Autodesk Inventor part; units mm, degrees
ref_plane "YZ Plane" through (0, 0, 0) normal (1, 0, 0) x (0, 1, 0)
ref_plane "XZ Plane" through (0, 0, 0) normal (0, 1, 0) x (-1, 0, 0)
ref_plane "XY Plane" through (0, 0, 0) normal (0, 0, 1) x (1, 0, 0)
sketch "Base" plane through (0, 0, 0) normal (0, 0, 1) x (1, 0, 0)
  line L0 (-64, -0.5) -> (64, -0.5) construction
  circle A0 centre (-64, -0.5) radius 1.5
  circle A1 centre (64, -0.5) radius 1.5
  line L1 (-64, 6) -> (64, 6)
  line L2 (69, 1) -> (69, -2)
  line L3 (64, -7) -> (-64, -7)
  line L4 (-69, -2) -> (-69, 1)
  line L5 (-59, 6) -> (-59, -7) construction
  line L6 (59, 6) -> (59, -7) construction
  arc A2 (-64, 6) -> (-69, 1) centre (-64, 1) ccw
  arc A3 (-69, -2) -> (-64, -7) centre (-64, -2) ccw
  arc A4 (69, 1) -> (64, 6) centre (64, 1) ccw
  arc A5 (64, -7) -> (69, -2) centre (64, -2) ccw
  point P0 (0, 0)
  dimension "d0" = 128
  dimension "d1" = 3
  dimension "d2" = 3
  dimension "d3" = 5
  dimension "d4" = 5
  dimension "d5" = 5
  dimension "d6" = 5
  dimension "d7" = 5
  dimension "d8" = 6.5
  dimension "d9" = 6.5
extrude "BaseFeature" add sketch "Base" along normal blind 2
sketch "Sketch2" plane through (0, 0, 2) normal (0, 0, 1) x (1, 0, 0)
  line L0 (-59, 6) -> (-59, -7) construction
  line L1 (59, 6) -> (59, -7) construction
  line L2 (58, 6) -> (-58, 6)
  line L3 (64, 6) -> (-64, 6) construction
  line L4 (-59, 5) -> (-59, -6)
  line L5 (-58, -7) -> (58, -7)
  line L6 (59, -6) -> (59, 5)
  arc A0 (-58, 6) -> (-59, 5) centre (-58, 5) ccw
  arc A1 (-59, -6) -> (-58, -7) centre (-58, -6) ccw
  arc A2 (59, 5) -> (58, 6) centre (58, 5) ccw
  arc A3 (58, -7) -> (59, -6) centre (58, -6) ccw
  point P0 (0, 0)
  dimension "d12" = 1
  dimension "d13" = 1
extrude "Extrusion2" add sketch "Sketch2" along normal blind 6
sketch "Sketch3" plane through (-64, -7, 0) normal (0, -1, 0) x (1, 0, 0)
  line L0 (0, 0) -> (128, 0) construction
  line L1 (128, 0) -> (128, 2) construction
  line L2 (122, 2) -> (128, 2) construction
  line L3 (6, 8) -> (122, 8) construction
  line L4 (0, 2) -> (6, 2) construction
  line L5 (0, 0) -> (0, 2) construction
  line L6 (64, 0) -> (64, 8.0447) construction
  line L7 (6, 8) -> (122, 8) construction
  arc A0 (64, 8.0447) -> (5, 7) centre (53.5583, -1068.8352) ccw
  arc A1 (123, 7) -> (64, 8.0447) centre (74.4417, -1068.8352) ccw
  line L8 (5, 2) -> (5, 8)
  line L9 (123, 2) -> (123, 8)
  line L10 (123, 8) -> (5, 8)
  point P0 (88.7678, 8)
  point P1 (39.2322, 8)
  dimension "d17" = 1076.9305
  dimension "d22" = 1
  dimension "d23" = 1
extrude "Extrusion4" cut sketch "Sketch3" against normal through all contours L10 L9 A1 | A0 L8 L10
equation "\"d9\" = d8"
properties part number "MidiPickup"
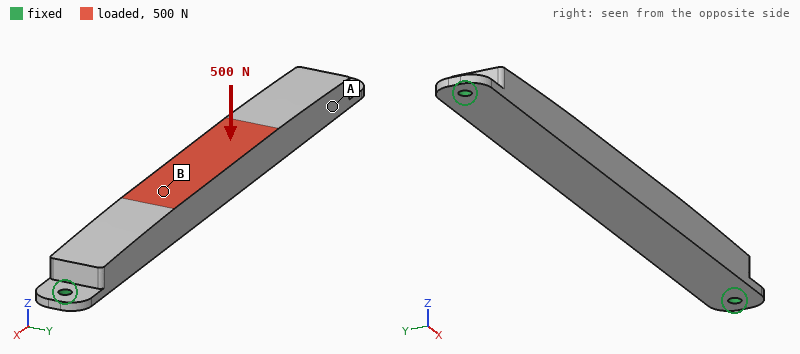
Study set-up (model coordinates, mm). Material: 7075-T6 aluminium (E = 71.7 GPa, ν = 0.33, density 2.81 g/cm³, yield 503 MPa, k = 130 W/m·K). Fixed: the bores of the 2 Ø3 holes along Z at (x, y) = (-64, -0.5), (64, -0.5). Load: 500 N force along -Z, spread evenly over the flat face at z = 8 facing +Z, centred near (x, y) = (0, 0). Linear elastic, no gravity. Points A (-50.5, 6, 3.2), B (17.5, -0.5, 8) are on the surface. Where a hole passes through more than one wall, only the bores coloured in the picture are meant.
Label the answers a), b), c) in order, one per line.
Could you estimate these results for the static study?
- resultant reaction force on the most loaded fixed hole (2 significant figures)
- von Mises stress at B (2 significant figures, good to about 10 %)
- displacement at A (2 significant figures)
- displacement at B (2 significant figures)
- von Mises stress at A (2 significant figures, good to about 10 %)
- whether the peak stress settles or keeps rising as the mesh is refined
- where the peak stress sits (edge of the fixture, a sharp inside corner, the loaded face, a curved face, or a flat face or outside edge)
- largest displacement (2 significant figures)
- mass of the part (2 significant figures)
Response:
a) 1.2 kN
b) 58 MPa
c) 0.062 mm
d) 0.23 mm
e) 17 MPa
f) keeps rising
g) edge of the fixture
h) 0.26 mm
i) 35 g
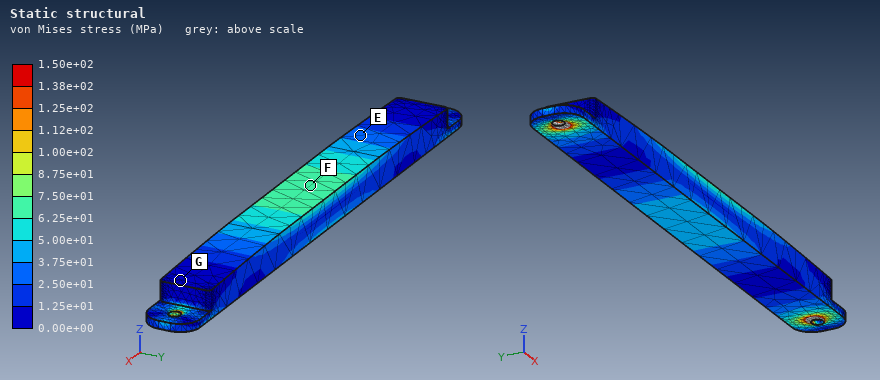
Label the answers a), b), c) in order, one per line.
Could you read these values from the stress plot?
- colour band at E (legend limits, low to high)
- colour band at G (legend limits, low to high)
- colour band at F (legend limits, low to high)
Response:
a) 2.50e+01 to 3.75e+01 MPa
b) 0.00e+00 to 1.25e+01 MPa
c) 6.25e+01 to 7.50e+01 MPa
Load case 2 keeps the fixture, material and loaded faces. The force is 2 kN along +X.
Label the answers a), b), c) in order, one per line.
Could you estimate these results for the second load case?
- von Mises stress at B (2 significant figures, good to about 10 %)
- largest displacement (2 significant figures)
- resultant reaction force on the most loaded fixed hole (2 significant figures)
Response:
a) 14 MPa
b) 14 µm
c) 1.0 kN
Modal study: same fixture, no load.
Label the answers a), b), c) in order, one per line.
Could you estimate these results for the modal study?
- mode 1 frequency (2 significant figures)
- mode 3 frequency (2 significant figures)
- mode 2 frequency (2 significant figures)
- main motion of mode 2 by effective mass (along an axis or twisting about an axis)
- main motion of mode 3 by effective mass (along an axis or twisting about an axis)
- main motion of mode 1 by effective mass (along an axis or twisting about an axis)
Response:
a) 1600 Hz
b) 4300 Hz
c) 2100 Hz
d) along Y
e) twisting about X
f) along Z
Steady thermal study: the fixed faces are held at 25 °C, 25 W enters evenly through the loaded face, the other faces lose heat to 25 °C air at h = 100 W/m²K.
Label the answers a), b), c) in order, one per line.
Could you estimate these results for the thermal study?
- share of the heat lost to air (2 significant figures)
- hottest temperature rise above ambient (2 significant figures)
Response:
a) 49 %
b) 43 K
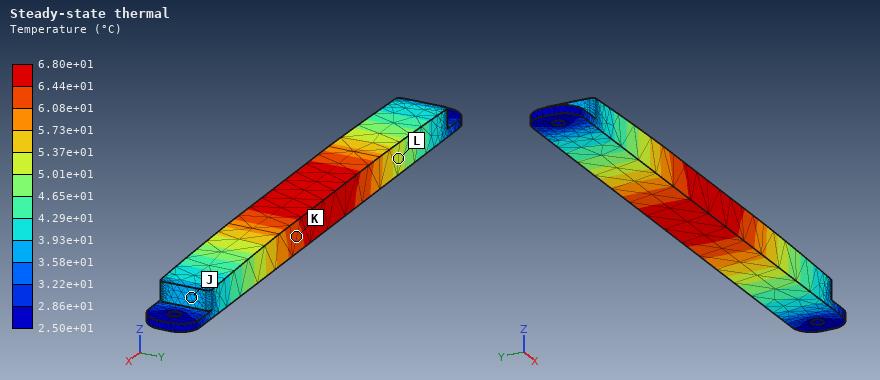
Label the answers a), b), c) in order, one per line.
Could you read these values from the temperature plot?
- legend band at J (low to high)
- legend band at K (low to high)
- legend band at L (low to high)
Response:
a) 3.58e+01 to 3.93e+01 °C
b) 6.08e+01 to 6.44e+01 °C
c) 5.01e+01 to 5.37e+01 °C
